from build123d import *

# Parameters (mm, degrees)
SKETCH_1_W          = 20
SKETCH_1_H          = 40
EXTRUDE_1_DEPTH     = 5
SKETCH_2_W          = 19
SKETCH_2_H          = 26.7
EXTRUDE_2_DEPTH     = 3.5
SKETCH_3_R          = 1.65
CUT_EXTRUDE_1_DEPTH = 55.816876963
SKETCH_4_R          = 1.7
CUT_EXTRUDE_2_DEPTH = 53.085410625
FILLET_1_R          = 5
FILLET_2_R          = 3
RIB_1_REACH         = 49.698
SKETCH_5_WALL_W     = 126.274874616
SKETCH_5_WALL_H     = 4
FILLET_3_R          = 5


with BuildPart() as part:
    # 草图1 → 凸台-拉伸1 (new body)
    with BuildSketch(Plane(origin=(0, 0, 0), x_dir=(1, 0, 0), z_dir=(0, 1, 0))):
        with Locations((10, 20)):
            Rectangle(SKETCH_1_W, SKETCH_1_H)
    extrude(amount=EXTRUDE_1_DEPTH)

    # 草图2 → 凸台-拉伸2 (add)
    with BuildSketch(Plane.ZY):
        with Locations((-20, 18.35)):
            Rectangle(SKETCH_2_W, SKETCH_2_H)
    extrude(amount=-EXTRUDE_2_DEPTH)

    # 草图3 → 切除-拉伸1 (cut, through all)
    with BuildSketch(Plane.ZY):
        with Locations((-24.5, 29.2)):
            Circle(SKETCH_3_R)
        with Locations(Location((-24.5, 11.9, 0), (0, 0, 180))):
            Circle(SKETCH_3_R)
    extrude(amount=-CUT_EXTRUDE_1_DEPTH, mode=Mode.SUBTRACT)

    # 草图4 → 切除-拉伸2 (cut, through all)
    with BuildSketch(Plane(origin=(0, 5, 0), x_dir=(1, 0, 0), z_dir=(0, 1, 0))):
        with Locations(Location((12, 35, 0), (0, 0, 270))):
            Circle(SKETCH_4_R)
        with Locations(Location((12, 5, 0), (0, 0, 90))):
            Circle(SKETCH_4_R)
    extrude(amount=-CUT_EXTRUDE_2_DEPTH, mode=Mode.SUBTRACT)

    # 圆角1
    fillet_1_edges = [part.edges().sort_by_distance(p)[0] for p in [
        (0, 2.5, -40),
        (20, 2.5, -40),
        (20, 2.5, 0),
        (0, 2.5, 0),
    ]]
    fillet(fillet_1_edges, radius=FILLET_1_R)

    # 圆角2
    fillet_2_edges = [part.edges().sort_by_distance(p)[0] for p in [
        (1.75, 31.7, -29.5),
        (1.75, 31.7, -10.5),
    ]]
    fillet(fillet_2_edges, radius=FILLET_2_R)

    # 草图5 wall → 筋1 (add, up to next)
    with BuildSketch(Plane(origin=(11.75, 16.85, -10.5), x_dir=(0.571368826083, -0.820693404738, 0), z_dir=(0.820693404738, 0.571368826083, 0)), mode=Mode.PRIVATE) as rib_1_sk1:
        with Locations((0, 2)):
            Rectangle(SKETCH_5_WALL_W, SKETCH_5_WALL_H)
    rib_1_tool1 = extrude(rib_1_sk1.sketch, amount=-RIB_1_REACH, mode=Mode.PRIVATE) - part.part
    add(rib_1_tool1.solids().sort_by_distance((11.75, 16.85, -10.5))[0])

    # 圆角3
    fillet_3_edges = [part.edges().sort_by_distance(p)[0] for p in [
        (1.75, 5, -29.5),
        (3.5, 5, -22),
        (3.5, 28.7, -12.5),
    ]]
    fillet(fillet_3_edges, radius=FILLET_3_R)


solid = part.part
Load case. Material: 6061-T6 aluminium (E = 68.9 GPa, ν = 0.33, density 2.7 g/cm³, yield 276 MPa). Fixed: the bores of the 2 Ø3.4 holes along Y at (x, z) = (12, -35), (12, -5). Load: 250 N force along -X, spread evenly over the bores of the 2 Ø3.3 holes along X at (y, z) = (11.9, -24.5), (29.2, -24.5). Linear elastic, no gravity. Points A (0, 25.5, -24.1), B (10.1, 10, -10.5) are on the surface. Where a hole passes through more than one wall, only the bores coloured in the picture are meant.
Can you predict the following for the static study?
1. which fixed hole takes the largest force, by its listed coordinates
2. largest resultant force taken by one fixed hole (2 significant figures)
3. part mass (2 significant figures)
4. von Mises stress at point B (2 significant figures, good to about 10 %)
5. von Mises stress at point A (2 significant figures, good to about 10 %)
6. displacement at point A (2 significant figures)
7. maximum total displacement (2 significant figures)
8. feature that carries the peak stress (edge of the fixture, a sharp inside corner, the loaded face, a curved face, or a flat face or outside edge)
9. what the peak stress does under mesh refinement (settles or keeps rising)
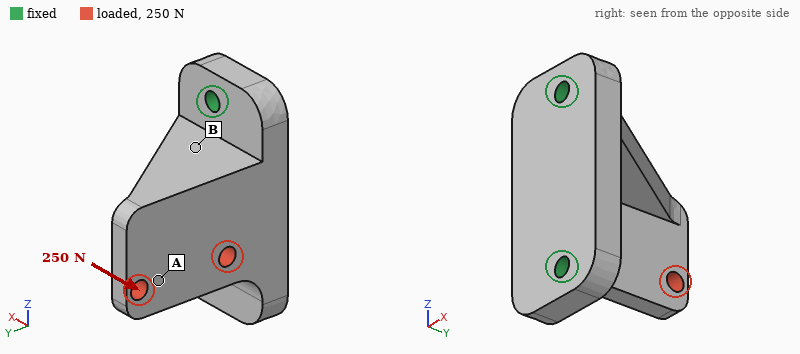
(12, -35)
160 N
17 g
8.8 MPa
27 MPa
65 µm
98 µm
edge of the fixture
keeps rising
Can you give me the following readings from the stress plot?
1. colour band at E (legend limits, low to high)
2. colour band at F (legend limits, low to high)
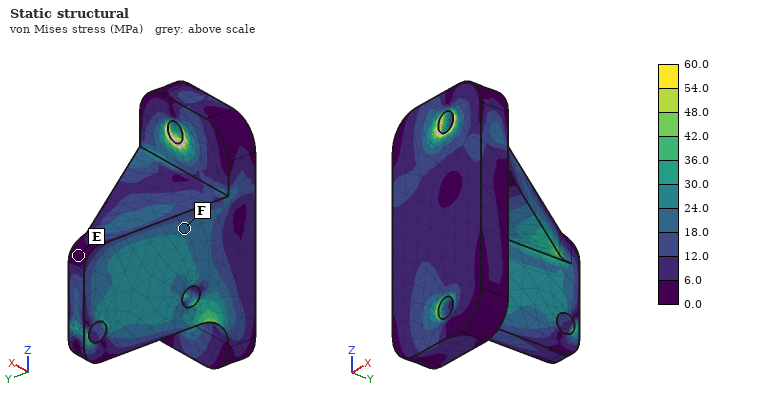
0.0 to 6.0 MPa
18.0 to 24.0 MPa
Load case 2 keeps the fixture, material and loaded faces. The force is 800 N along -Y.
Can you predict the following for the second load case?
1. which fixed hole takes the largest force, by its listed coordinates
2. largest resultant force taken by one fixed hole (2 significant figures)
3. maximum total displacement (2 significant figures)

(12, -35)
540 N
63 µm
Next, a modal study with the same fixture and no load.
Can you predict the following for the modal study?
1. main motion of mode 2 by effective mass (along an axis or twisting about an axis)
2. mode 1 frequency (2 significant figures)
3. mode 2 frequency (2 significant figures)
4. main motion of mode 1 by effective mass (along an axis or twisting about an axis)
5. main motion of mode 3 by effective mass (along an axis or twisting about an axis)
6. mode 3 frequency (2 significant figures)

along Z
5600 Hz
10 kHz
along X
along Y
13 kHz
